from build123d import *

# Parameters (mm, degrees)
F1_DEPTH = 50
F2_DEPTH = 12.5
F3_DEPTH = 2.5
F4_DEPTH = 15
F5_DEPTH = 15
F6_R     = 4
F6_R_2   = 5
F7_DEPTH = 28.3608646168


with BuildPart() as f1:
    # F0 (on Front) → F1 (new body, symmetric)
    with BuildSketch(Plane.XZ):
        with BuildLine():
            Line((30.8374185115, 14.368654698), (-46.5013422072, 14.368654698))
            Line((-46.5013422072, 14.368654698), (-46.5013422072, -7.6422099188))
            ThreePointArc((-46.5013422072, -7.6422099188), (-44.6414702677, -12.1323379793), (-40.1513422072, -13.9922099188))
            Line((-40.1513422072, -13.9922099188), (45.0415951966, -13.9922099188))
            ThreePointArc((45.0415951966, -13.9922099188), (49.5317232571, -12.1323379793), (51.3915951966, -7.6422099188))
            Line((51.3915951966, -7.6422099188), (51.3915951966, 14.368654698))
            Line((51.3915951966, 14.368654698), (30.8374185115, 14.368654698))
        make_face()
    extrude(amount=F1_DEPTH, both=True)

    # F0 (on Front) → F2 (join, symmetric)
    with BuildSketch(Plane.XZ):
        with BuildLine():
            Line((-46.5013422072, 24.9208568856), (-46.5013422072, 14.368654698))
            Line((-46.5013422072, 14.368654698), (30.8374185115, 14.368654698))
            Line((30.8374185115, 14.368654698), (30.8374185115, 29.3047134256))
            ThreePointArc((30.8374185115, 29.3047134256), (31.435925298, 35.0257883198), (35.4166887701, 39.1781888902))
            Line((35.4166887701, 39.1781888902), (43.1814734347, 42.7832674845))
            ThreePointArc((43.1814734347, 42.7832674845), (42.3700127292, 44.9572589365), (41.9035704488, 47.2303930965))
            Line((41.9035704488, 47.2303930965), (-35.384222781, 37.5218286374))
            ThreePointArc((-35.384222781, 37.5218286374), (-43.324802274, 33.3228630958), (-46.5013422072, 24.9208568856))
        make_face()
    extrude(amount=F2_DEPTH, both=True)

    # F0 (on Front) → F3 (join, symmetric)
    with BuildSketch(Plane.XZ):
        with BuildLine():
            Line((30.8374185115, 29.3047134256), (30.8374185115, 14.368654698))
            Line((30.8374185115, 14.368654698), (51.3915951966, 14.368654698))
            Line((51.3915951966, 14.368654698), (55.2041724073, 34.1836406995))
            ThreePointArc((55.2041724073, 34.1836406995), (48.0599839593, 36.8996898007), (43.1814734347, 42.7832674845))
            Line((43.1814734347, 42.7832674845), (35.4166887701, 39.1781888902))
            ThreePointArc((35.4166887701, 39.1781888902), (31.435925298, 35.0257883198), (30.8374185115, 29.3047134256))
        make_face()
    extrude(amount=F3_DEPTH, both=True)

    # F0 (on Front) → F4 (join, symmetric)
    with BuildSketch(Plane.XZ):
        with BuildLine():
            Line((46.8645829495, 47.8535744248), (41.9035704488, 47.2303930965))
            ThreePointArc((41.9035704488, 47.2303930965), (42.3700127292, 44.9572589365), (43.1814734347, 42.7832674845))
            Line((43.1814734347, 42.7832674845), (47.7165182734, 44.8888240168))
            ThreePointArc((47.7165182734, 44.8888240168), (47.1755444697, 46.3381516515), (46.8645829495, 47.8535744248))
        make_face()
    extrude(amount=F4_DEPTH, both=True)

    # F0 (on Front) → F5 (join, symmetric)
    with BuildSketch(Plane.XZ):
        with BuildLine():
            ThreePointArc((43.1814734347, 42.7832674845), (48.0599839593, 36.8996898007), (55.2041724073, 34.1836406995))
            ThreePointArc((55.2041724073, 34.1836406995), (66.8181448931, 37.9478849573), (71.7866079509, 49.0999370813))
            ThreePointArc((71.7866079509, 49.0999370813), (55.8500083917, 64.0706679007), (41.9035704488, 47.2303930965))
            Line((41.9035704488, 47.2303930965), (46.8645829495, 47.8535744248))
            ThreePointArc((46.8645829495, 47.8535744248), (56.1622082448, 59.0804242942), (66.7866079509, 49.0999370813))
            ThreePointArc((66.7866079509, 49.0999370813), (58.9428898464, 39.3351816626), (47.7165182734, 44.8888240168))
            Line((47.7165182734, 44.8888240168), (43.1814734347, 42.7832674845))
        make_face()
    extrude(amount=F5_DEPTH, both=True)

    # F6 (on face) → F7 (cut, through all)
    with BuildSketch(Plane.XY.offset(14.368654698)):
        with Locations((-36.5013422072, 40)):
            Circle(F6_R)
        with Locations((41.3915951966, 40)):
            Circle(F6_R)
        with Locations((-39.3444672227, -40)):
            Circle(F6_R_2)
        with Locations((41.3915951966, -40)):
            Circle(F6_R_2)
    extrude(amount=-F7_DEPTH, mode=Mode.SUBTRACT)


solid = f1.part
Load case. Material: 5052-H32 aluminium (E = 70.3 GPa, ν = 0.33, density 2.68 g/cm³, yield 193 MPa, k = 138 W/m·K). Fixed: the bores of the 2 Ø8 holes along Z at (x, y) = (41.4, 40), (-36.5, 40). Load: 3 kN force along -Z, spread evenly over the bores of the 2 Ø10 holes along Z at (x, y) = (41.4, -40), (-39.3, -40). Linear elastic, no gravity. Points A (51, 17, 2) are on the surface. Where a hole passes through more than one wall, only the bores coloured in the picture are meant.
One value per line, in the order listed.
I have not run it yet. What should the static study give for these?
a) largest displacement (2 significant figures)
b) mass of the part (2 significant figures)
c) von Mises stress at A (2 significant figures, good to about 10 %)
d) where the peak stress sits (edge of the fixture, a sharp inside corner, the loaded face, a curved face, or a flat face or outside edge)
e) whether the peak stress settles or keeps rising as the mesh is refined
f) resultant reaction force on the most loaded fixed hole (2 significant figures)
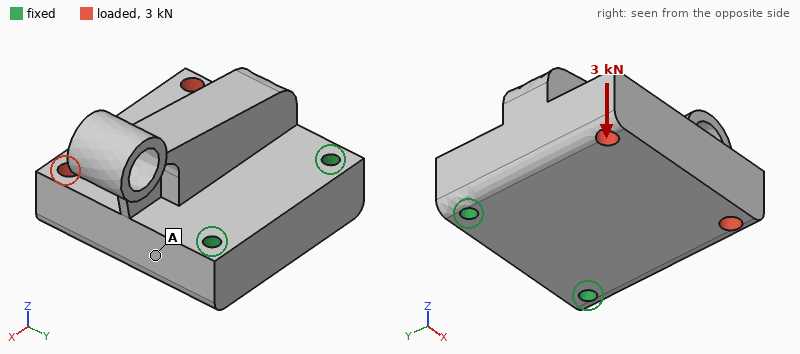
75 µm
900 g
7.8 MPa
edge of the fixture
keeps rising
1.5 kN
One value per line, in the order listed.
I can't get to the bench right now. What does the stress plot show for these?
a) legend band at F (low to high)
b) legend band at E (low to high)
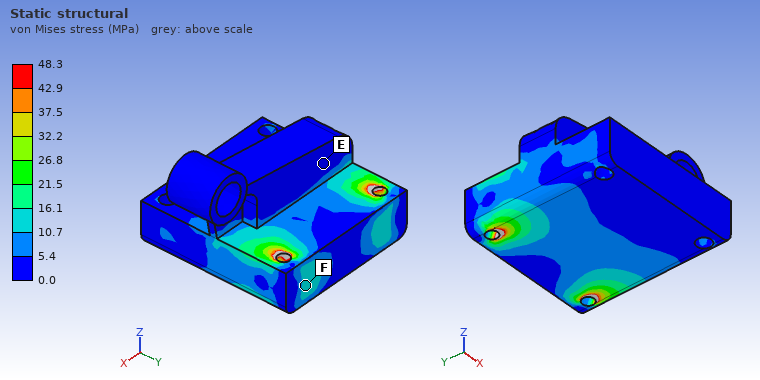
10.7 to 16.1 MPa
0.0 to 5.4 MPa
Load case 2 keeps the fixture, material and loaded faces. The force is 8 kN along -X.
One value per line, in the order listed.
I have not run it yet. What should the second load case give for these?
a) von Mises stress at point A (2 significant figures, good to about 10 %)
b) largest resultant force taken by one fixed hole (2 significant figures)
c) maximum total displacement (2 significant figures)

10 MPa
8.9 kN
27 µm
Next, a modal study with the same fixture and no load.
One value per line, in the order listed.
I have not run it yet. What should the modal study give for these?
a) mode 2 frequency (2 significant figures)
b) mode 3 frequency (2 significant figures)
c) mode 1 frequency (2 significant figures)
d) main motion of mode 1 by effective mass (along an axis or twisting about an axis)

3700 Hz
4200 Hz
2000 Hz
along Z
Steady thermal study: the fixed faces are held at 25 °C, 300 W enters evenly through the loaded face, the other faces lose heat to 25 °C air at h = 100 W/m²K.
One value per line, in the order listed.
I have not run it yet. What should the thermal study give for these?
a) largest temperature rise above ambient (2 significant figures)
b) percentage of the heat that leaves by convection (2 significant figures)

76 K
36 %
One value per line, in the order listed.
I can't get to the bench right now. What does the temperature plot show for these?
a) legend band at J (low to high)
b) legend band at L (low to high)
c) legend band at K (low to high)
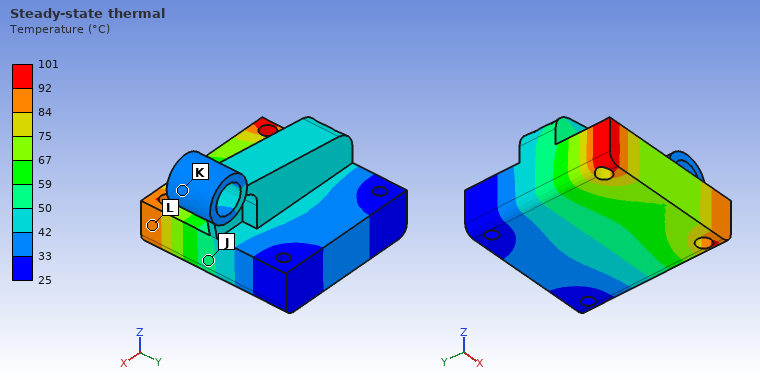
50 to 59 °C
84 to 92 °C
33 to 42 °C
